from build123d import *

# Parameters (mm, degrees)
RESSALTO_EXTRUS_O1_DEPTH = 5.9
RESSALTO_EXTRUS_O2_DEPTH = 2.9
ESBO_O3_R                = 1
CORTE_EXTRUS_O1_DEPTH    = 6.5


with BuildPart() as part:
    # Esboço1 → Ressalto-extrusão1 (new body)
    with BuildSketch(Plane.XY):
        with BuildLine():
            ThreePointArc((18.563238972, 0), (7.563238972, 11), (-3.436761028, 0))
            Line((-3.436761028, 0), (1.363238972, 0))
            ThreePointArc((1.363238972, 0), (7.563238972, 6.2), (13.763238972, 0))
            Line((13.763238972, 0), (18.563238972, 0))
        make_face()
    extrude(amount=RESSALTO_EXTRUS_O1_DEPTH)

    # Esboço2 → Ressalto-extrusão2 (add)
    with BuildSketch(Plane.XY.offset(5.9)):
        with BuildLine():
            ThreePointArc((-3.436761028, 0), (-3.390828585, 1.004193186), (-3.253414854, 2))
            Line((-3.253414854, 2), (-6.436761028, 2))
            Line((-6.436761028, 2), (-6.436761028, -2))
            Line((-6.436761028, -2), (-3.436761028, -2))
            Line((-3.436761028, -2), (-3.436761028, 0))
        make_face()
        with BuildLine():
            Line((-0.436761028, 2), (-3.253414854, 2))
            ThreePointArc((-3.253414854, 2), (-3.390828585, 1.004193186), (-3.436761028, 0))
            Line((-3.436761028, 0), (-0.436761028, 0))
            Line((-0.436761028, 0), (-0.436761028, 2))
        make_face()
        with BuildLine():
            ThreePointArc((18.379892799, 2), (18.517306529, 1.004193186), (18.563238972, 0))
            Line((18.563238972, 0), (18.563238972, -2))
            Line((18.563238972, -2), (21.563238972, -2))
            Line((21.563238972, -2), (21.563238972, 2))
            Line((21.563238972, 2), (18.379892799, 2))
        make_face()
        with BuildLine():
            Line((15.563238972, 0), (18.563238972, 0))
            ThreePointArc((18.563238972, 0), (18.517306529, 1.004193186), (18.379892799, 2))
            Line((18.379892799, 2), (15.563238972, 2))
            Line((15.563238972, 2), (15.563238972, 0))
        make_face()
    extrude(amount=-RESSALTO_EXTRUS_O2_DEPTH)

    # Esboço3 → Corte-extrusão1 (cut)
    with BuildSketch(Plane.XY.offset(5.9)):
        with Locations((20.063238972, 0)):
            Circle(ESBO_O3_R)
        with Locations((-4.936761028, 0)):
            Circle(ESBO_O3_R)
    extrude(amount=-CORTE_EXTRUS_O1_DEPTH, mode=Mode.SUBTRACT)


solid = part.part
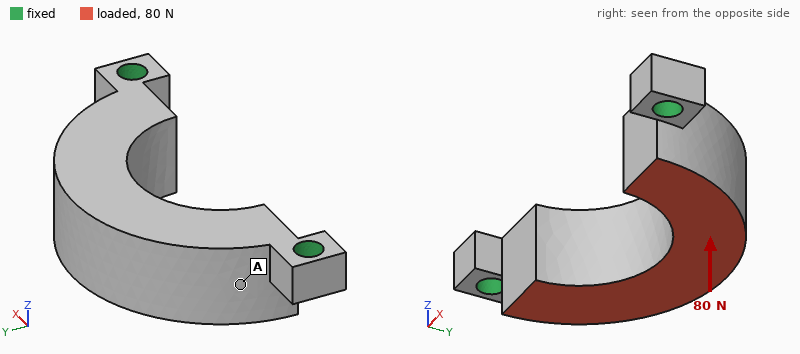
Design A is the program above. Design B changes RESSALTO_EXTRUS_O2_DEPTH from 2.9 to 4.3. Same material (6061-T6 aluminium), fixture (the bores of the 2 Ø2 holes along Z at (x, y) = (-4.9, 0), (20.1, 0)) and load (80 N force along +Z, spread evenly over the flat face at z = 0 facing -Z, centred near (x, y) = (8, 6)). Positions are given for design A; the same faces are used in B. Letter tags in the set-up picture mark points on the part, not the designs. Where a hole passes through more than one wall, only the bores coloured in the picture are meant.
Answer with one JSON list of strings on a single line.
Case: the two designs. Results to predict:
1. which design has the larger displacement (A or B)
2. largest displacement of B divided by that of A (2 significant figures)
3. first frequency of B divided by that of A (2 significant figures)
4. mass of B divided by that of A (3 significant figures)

["A", "0.44", "1.5", "1.03"]
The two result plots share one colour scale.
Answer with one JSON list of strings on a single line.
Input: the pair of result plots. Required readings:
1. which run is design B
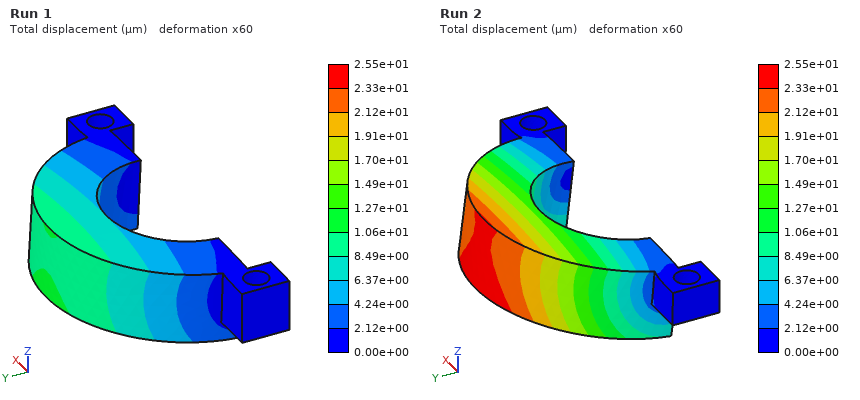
["Run 1"]
